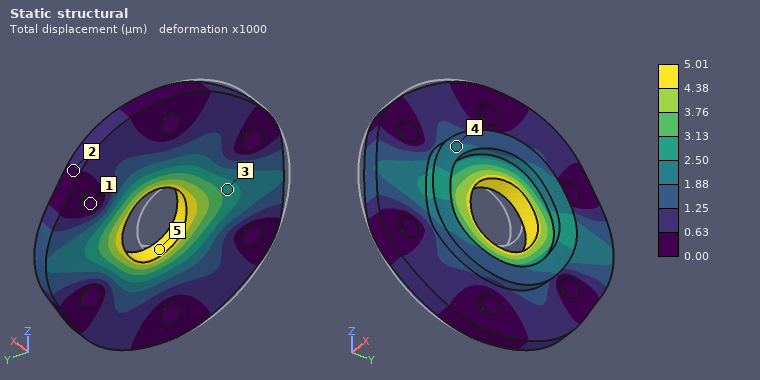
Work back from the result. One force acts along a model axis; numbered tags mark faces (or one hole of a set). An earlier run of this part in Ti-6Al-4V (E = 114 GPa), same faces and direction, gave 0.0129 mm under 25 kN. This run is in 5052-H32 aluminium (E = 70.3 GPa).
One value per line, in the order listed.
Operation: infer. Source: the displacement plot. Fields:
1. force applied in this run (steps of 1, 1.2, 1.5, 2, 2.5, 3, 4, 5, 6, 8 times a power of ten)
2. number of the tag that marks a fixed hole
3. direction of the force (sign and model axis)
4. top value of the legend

6 kN
1
+Y
5.01 µm
